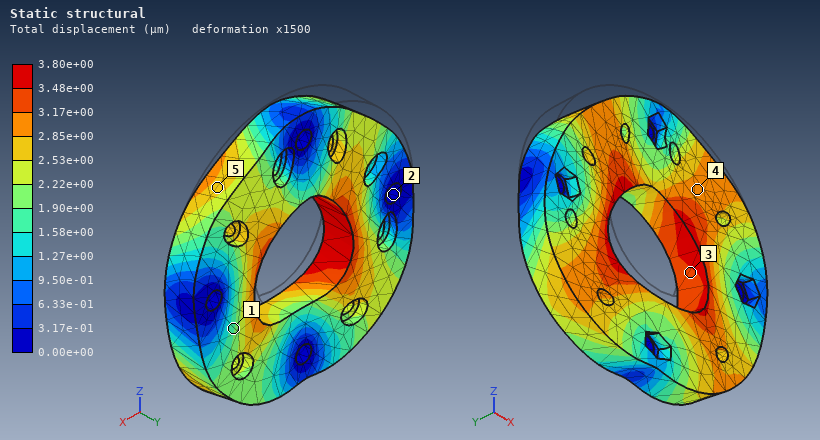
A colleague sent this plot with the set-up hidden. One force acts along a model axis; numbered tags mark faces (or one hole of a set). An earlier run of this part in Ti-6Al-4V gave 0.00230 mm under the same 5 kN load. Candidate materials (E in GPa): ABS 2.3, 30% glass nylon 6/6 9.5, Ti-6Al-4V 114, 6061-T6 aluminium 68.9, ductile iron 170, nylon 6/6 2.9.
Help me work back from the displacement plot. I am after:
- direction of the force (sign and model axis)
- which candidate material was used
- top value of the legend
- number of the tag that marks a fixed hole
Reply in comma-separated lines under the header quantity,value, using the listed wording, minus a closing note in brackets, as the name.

quantity,value
direction of the force,-Z
which candidate material was used,6061-T6 aluminium
top value of the legend,3.80e+00 µm
number of the tag that marks a fixed hole,2
